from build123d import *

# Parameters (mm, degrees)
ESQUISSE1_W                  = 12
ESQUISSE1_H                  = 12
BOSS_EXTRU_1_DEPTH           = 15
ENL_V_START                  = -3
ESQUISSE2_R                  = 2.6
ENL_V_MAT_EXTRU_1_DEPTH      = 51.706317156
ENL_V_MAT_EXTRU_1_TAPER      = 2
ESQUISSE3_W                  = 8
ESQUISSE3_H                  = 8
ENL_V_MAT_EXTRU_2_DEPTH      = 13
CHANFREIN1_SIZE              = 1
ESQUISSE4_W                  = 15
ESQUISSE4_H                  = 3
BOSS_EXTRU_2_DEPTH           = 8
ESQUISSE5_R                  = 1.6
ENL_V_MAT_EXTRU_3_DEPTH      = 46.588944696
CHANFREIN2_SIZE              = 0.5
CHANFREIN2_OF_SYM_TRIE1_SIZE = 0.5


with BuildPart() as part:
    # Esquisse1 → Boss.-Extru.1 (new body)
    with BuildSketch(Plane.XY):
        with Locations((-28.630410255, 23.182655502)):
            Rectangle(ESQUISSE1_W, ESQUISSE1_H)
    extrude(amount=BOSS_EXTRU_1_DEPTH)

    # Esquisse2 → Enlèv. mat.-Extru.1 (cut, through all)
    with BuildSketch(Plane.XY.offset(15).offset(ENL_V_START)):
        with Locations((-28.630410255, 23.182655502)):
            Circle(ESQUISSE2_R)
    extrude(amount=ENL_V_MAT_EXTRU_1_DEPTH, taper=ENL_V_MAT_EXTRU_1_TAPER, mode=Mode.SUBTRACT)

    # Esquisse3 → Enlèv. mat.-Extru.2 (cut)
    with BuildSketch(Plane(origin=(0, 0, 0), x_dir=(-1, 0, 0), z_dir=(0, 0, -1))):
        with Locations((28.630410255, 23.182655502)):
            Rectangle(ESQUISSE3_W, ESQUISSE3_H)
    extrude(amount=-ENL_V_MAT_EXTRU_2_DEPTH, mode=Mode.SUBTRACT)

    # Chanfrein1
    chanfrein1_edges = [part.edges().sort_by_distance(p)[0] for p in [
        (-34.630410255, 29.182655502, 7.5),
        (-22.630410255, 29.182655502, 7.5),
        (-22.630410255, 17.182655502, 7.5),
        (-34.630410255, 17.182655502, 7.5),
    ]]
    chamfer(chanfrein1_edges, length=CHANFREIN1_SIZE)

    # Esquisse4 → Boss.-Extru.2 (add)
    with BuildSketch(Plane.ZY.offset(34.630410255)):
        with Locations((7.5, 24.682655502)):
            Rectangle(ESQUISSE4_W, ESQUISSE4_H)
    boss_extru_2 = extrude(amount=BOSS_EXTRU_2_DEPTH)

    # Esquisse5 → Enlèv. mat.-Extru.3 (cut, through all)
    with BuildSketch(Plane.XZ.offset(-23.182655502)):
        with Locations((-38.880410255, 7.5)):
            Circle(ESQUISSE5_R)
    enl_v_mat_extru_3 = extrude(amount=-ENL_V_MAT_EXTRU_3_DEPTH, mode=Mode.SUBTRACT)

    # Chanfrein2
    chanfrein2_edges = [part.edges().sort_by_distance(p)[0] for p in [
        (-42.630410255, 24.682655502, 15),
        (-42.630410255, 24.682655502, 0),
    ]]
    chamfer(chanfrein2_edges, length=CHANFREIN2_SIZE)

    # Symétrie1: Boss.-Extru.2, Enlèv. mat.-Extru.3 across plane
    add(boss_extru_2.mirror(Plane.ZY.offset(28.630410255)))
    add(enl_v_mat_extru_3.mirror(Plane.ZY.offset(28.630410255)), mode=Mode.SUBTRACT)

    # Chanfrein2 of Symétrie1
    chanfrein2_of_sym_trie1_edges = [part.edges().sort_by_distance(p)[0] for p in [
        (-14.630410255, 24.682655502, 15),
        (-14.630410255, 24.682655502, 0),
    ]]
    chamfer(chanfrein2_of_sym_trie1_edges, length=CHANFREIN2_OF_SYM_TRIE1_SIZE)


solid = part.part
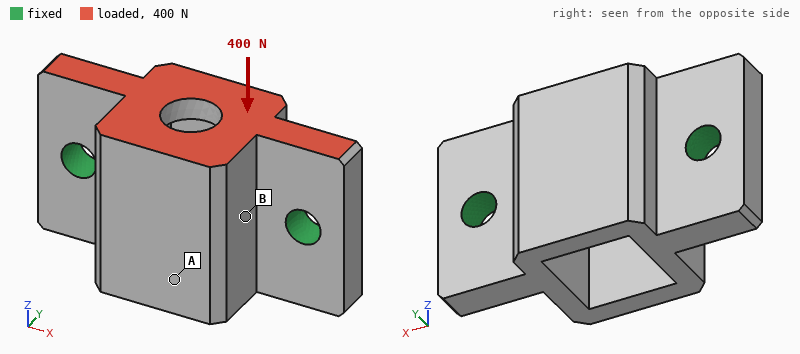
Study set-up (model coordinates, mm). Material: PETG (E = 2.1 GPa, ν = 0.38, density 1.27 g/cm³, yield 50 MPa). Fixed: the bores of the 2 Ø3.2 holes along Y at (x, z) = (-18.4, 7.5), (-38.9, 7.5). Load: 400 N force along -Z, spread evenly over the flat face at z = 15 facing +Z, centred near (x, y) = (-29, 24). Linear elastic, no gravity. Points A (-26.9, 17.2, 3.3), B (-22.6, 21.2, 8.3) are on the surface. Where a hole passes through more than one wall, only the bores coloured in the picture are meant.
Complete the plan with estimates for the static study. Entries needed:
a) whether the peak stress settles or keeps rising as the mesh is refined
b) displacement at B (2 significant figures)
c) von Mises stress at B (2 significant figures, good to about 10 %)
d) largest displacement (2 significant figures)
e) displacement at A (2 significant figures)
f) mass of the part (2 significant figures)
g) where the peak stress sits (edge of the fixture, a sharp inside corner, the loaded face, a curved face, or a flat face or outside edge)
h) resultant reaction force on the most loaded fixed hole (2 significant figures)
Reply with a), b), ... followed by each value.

a) keeps rising
b) 0.072 mm
c) 6.3 MPa
d) 0.14 mm
e) 0.12 mm
f) 2.4 g
g) edge of the fixture
h) 200 N
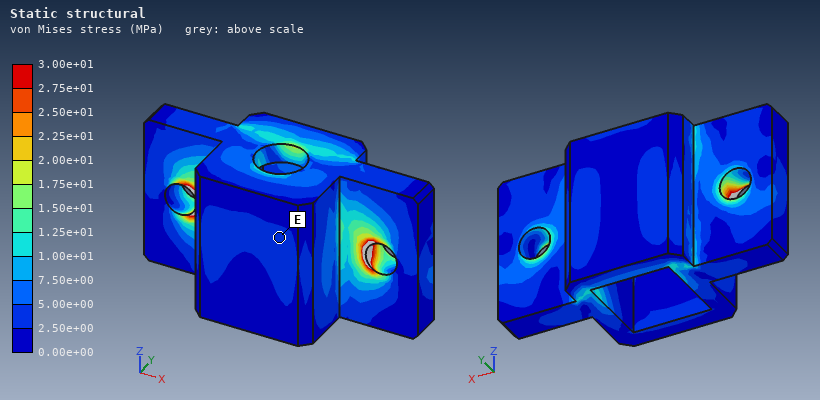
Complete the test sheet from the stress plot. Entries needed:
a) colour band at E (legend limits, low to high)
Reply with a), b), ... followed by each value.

a) 2.50e+00 to 5.00e+00 MPa
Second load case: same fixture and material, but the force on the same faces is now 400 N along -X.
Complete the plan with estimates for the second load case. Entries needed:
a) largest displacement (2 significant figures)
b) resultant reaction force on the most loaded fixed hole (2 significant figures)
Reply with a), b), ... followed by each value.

a) 0.11 mm
b) 240 N
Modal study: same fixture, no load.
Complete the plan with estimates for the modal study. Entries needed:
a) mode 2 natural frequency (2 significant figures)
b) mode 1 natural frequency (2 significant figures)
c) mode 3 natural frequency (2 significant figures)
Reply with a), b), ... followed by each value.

a) 8000 Hz
b) 4400 Hz
c) 8100 Hz
